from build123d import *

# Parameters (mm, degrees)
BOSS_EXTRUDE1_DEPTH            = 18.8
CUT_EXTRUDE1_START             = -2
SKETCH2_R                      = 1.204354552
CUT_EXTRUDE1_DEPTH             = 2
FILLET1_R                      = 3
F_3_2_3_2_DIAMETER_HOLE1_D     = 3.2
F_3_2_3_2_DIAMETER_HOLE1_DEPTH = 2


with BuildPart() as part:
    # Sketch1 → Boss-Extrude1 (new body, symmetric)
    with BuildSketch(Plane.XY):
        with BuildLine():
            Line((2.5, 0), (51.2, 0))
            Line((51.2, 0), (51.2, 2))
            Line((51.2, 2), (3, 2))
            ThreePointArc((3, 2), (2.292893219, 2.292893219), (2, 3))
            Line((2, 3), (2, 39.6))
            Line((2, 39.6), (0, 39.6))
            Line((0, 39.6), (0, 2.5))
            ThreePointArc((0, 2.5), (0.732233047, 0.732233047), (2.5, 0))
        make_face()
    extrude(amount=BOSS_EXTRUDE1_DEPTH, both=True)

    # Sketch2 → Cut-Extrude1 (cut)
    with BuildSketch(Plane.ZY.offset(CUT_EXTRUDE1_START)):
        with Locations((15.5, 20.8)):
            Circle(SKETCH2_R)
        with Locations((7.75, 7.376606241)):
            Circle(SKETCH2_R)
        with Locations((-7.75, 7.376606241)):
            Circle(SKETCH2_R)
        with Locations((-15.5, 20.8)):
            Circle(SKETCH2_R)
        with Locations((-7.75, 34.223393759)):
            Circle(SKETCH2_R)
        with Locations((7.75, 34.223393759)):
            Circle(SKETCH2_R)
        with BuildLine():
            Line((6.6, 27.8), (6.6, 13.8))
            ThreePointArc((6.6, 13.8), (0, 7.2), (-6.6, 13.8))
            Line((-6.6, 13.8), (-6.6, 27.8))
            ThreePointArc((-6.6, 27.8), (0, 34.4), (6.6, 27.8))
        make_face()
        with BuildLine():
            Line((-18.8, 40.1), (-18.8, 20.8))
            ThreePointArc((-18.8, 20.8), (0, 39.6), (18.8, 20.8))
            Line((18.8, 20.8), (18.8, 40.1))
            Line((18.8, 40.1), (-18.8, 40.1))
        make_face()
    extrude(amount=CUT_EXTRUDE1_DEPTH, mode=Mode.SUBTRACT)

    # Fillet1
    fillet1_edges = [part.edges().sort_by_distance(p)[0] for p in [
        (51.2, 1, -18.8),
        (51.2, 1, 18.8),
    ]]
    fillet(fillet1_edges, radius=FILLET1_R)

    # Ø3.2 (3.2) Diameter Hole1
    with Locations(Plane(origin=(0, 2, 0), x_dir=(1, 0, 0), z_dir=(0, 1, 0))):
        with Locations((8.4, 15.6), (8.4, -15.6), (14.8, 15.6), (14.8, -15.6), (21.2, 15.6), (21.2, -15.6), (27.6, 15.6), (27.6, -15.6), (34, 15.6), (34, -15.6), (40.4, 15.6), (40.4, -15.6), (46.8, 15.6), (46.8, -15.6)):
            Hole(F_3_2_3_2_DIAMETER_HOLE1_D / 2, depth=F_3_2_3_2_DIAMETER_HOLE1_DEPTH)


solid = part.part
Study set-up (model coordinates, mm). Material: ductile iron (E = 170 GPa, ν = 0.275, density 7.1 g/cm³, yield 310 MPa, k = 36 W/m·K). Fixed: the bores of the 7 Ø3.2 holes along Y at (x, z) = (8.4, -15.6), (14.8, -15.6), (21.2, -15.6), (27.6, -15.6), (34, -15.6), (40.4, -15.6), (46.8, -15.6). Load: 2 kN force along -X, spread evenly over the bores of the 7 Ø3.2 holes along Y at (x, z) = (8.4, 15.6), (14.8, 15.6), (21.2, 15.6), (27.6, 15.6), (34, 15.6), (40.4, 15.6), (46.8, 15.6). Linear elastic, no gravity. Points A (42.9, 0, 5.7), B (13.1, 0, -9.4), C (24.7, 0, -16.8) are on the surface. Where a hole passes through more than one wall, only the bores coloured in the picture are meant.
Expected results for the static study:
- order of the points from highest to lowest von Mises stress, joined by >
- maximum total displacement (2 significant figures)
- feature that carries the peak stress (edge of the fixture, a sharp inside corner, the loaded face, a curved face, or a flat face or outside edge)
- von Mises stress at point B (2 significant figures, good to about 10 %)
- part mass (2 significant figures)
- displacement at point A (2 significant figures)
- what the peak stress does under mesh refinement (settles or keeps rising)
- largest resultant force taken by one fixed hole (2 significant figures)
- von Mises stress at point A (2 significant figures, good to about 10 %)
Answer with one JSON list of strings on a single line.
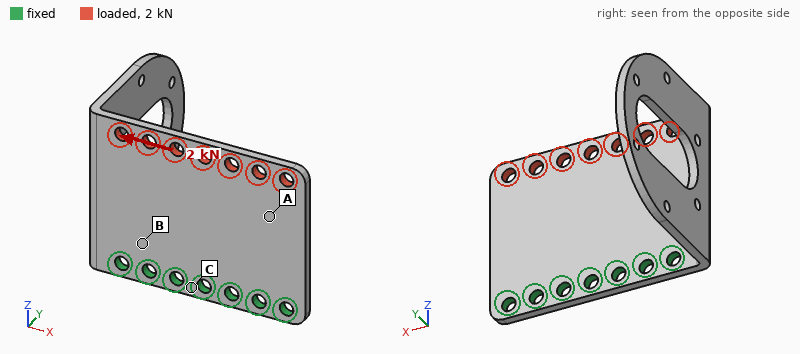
["B > A > C", "22 µm", "edge of the fixture", "58 MPa", "38 g", "12 µm", "keeps rising", "1.3 kN", "33 MPa"]
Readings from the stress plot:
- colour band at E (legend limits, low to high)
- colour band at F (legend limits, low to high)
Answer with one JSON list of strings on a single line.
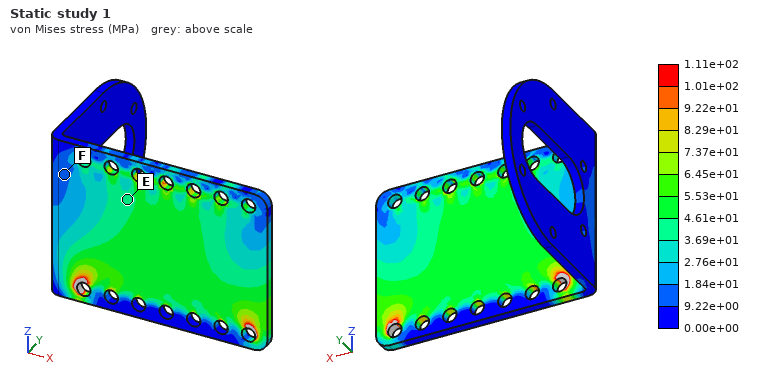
["3.69e+01 to 4.61e+01 MPa", "9.22e+00 to 1.84e+01 MPa"]
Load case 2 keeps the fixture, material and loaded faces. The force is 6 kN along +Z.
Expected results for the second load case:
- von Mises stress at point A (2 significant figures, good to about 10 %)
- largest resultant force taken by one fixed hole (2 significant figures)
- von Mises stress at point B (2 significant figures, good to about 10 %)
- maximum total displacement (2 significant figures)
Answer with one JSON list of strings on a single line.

["65 MPa", "1.1 kN", "61 MPa", "14 µm"]
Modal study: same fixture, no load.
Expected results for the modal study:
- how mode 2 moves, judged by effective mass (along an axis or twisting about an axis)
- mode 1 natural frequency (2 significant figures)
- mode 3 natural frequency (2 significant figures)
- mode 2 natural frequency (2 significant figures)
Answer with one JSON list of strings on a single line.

["along Y", "870 Hz", "2100 Hz", "1200 Hz"]
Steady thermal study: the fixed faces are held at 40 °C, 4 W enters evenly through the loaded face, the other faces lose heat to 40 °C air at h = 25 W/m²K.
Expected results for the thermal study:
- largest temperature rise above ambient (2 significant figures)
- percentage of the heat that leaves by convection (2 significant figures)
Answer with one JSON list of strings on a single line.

["29 K", "35 %"]
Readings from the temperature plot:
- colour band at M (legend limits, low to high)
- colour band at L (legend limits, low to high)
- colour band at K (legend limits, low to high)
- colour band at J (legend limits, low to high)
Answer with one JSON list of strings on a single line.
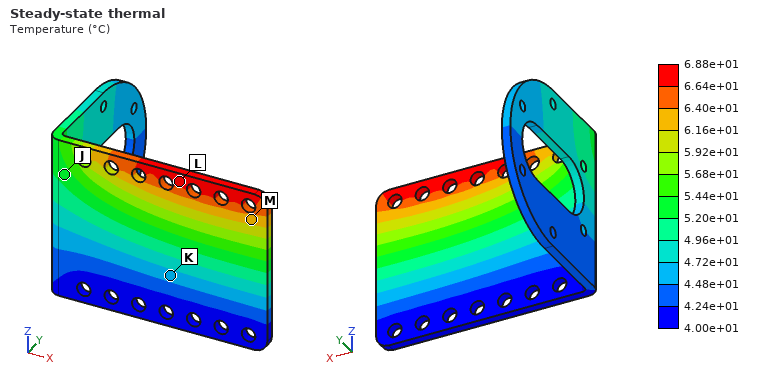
["6.16e+01 to 6.40e+01 °C", "6.64e+01 to 6.88e+01 °C", "4.48e+01 to 4.72e+01 °C", "5.20e+01 to 5.44e+01 °C"]
